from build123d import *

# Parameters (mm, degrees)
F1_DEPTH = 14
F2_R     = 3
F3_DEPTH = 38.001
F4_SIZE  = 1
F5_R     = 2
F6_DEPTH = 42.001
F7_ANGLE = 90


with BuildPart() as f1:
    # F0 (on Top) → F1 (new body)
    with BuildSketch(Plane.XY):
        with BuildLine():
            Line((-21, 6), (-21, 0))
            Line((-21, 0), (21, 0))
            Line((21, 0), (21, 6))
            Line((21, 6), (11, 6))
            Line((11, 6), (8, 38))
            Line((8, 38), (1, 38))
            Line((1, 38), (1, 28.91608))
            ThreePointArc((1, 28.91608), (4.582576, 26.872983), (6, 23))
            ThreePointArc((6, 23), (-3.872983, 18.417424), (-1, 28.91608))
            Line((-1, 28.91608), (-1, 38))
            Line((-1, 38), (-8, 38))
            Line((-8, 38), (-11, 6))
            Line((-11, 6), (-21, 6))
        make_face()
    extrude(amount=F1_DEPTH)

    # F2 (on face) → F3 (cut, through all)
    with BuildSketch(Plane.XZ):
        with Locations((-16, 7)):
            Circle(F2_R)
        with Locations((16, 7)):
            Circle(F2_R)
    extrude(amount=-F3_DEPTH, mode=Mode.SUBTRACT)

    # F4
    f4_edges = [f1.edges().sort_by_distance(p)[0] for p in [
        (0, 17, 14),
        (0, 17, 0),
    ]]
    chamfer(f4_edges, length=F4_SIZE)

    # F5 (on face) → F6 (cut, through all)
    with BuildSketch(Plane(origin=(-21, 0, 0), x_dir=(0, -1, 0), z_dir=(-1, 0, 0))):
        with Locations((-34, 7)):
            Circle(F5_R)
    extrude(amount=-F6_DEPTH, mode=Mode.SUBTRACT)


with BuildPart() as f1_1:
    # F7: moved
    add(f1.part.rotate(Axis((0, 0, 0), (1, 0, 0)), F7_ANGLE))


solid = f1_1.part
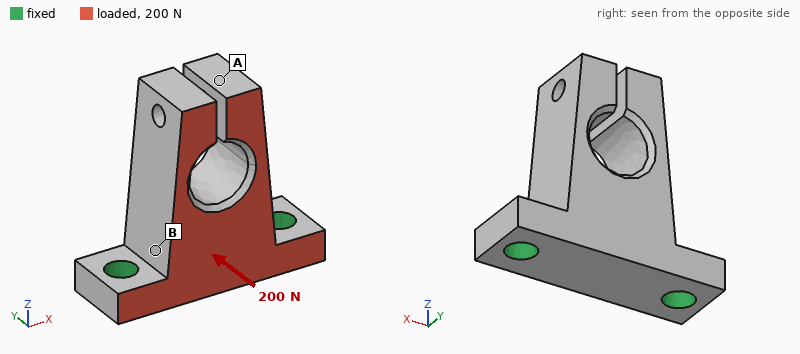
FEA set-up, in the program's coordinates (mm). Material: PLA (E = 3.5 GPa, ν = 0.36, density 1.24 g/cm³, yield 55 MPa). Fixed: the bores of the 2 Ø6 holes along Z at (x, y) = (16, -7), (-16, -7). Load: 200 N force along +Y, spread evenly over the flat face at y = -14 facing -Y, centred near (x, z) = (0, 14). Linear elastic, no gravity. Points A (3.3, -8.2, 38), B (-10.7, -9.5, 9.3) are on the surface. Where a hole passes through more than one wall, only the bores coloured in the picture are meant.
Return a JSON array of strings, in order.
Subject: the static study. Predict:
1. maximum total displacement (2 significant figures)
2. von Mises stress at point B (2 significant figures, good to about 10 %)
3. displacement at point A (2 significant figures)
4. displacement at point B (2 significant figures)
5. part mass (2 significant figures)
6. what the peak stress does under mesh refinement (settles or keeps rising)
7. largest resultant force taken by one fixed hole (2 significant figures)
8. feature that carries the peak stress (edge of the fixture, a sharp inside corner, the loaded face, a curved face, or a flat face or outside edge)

["0.23 mm", "3.0 MPa", "0.23 mm", "0.038 mm", "12 g", "keeps rising", "100 N", "edge of the fixture"]
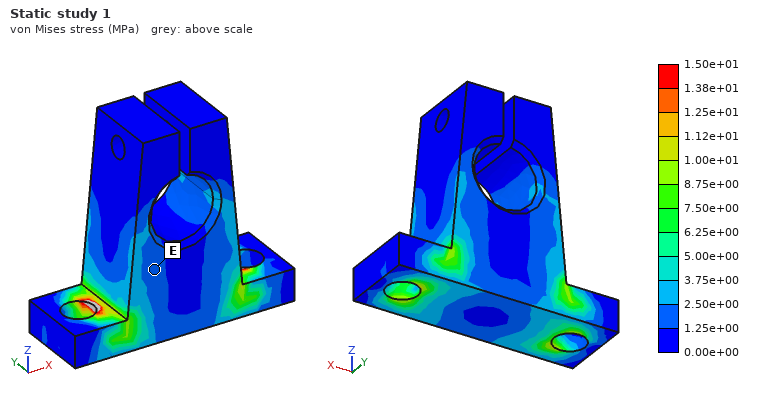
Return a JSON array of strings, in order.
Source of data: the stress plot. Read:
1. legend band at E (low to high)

["1.25e+00 to 2.50e+00 MPa"]
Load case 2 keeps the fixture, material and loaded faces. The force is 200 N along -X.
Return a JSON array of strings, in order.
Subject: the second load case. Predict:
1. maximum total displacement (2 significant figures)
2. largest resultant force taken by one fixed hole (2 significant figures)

["0.25 mm", "140 N"]
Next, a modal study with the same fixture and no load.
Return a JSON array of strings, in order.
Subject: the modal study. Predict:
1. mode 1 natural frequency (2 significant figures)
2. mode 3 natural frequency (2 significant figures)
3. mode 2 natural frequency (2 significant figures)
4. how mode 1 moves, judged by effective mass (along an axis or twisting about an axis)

["1700 Hz", "1800 Hz", "1800 Hz", "along Y"]
